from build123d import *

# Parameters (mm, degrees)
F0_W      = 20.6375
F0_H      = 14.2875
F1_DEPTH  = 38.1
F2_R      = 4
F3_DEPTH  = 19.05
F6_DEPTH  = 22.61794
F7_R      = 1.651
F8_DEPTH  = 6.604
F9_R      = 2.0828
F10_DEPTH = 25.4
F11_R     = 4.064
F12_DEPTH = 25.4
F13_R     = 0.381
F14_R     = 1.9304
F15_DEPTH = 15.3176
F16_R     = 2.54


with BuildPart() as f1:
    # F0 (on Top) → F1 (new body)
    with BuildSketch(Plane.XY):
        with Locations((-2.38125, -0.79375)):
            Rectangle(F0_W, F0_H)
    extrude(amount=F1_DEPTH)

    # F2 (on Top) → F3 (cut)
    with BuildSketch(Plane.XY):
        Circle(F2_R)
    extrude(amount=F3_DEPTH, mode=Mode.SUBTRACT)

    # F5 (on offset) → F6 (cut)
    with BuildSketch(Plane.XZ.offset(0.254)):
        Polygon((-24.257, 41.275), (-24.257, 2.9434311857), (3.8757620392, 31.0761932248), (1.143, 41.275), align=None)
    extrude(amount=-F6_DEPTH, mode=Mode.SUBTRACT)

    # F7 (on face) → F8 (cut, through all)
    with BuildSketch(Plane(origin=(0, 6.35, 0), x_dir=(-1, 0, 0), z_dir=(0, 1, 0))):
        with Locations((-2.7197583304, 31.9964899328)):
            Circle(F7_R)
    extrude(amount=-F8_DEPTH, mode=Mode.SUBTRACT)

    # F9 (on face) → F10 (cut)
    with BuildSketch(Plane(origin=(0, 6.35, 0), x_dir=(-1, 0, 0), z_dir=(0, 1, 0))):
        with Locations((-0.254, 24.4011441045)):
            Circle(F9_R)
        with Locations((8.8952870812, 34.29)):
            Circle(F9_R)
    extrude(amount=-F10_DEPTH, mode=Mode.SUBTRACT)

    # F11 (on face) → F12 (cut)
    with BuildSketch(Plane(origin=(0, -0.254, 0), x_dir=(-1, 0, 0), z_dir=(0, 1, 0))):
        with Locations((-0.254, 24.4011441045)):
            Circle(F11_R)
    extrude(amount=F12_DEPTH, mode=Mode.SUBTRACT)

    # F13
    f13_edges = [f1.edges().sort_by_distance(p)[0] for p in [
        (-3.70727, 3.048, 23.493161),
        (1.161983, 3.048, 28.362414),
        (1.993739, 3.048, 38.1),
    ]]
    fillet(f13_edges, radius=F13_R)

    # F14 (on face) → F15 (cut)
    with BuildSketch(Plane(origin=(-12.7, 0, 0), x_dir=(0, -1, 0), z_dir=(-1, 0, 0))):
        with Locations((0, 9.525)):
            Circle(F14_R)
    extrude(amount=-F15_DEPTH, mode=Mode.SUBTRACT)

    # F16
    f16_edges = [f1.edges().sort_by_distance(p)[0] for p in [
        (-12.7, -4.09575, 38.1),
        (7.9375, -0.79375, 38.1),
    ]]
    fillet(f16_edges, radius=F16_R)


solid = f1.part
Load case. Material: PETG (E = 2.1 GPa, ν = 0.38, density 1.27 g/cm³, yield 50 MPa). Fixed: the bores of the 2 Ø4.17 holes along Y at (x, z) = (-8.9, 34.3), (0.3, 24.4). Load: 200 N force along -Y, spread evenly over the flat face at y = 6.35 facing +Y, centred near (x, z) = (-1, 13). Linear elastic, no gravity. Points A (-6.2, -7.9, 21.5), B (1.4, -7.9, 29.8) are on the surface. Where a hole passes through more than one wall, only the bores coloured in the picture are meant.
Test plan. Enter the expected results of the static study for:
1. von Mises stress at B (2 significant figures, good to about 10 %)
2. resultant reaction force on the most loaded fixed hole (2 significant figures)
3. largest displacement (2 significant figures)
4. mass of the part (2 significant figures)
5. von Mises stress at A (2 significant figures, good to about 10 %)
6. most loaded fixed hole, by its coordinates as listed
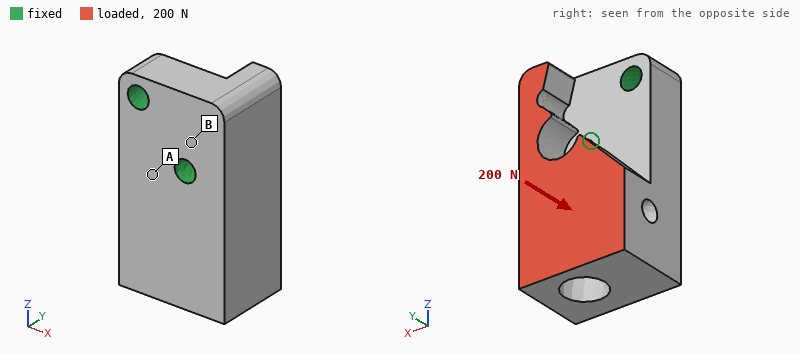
1.8 MPa
230 N
0.22 mm
10 g
4.3 MPa
(0.3, 24.4)
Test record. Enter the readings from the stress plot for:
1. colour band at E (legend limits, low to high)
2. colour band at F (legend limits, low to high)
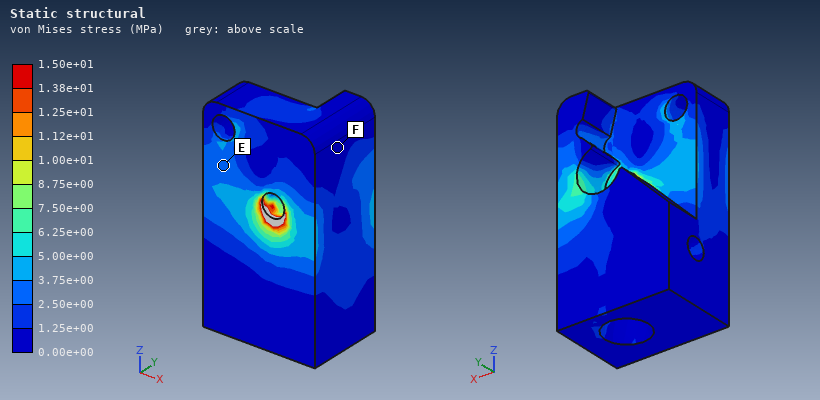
2.50e+00 to 3.75e+00 MPa
0.00e+00 to 1.25e+00 MPa
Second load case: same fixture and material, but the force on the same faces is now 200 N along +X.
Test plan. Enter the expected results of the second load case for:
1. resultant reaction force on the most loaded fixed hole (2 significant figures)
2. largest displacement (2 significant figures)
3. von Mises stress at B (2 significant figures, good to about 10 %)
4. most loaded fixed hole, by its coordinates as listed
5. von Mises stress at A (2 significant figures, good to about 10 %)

280 N
0.17 mm
2.1 MPa
(0.3, 24.4)
2.5 MPa
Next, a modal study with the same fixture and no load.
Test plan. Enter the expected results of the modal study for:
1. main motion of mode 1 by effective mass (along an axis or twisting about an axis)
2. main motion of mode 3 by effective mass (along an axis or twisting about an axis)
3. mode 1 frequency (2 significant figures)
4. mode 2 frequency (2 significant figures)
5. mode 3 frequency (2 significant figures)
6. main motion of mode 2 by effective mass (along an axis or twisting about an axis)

along Y
twisting about Z
2100 Hz
3100 Hz
4400 Hz
along X
